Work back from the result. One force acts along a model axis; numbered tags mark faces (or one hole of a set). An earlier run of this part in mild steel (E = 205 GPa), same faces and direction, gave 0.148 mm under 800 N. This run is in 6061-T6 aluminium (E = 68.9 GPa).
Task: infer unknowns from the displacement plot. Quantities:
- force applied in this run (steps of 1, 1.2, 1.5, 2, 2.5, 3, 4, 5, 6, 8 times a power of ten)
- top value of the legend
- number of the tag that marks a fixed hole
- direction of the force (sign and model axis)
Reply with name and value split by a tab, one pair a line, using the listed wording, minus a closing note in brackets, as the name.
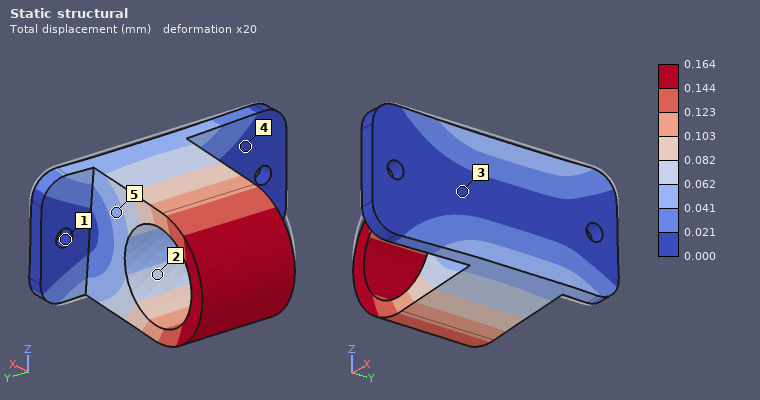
force applied in this run	300 N
top value of the legend	0.164 mm
number of the tag that marks a fixed hole	1
direction of the force	-Z
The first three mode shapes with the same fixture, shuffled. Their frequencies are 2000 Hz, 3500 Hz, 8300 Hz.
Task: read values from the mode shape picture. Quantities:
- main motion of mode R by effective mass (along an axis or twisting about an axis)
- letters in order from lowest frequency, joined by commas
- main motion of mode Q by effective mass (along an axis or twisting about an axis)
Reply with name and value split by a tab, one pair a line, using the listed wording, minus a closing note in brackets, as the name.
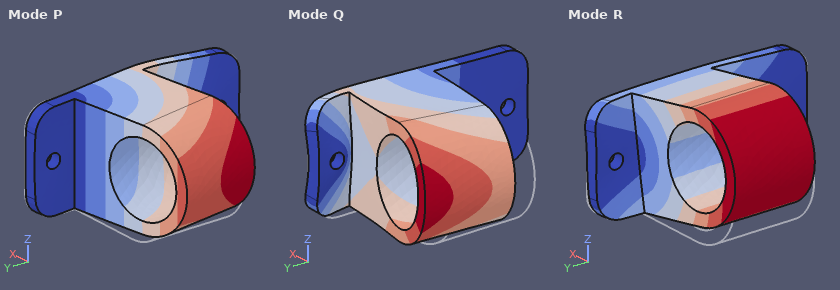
main motion of mode R by effective mass	along Z
letters in order from lowest frequency, joined by commas	R, P, Q
main motion of mode Q by effective mass	along X
